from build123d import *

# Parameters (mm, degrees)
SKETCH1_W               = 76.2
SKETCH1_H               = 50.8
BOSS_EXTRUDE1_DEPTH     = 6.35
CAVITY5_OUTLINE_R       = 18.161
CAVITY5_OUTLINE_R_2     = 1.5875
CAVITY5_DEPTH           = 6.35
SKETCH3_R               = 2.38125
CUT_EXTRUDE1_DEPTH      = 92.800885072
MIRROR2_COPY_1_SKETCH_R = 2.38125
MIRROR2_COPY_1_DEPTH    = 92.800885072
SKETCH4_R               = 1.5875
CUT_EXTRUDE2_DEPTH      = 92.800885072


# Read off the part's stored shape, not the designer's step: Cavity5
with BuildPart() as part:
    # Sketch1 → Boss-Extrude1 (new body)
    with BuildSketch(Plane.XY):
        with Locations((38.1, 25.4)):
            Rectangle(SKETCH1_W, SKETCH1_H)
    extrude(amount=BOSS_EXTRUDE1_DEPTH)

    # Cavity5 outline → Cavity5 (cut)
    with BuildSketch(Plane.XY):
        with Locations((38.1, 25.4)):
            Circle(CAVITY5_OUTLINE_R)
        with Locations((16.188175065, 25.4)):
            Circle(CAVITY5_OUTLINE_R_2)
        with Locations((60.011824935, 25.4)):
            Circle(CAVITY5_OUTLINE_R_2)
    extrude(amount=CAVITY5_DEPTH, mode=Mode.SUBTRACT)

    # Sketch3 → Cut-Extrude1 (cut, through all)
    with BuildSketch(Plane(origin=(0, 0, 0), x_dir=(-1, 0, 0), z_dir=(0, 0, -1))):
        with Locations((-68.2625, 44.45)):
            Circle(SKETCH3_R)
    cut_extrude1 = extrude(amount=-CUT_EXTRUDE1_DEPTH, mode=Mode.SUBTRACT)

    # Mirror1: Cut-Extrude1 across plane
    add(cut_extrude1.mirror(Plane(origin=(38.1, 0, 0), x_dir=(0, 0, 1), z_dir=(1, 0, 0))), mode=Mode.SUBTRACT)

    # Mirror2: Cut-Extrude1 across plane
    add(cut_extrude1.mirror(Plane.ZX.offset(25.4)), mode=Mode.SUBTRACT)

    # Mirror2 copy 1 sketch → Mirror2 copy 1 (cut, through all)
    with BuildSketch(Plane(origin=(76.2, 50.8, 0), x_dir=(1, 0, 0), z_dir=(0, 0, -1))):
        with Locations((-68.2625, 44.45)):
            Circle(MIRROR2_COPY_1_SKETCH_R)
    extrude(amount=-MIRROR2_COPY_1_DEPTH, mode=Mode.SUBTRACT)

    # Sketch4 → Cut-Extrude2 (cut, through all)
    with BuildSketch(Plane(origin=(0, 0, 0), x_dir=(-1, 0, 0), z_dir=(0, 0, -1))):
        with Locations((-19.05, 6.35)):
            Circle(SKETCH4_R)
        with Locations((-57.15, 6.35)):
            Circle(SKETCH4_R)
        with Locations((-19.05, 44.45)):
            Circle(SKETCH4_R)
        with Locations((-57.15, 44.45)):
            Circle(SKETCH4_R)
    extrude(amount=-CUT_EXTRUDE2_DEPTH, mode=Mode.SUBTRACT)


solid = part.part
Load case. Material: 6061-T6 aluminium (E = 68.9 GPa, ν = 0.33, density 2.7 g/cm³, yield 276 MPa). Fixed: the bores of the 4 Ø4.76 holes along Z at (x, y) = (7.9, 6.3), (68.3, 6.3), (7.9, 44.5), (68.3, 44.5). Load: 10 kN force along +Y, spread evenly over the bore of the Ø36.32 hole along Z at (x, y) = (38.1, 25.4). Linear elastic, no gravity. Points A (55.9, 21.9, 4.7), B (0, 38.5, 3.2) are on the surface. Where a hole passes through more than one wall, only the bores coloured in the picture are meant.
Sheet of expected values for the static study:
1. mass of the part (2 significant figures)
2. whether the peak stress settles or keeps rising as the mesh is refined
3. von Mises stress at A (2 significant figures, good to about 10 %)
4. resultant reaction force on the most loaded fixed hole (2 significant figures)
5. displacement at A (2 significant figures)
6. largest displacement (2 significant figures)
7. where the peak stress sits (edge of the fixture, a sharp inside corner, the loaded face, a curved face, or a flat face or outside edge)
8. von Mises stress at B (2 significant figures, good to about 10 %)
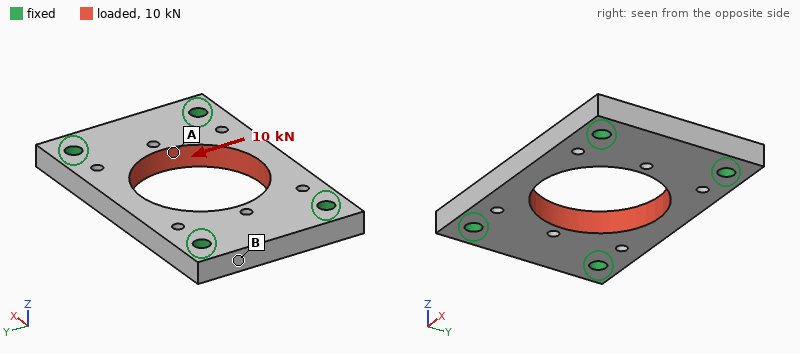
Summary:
47 g
keeps rising
35 MPa
2.7 kN
11 µm
36 µm
edge of the fixture
12 MPa
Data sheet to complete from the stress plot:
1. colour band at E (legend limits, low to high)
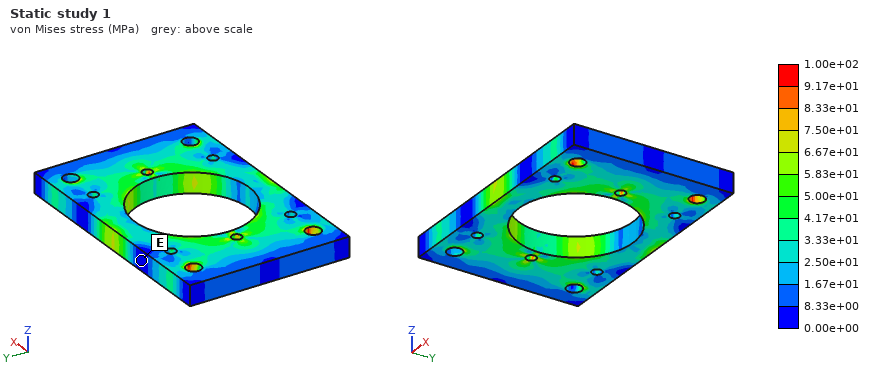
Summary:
0.00e+00 to 8.33e+00 MPa
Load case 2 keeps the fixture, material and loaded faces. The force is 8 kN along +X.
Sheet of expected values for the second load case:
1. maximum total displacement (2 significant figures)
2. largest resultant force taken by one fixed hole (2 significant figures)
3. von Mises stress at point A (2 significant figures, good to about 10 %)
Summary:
7.7 µm
2.0 kN
13 MPa
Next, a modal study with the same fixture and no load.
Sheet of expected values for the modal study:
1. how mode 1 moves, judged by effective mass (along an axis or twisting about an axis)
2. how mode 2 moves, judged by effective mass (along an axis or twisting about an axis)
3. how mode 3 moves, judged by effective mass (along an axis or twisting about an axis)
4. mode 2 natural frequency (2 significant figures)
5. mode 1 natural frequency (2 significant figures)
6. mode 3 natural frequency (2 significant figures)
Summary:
along Z
twisting about X
twisting about Y
11 kHz
10000 Hz
17 kHz
